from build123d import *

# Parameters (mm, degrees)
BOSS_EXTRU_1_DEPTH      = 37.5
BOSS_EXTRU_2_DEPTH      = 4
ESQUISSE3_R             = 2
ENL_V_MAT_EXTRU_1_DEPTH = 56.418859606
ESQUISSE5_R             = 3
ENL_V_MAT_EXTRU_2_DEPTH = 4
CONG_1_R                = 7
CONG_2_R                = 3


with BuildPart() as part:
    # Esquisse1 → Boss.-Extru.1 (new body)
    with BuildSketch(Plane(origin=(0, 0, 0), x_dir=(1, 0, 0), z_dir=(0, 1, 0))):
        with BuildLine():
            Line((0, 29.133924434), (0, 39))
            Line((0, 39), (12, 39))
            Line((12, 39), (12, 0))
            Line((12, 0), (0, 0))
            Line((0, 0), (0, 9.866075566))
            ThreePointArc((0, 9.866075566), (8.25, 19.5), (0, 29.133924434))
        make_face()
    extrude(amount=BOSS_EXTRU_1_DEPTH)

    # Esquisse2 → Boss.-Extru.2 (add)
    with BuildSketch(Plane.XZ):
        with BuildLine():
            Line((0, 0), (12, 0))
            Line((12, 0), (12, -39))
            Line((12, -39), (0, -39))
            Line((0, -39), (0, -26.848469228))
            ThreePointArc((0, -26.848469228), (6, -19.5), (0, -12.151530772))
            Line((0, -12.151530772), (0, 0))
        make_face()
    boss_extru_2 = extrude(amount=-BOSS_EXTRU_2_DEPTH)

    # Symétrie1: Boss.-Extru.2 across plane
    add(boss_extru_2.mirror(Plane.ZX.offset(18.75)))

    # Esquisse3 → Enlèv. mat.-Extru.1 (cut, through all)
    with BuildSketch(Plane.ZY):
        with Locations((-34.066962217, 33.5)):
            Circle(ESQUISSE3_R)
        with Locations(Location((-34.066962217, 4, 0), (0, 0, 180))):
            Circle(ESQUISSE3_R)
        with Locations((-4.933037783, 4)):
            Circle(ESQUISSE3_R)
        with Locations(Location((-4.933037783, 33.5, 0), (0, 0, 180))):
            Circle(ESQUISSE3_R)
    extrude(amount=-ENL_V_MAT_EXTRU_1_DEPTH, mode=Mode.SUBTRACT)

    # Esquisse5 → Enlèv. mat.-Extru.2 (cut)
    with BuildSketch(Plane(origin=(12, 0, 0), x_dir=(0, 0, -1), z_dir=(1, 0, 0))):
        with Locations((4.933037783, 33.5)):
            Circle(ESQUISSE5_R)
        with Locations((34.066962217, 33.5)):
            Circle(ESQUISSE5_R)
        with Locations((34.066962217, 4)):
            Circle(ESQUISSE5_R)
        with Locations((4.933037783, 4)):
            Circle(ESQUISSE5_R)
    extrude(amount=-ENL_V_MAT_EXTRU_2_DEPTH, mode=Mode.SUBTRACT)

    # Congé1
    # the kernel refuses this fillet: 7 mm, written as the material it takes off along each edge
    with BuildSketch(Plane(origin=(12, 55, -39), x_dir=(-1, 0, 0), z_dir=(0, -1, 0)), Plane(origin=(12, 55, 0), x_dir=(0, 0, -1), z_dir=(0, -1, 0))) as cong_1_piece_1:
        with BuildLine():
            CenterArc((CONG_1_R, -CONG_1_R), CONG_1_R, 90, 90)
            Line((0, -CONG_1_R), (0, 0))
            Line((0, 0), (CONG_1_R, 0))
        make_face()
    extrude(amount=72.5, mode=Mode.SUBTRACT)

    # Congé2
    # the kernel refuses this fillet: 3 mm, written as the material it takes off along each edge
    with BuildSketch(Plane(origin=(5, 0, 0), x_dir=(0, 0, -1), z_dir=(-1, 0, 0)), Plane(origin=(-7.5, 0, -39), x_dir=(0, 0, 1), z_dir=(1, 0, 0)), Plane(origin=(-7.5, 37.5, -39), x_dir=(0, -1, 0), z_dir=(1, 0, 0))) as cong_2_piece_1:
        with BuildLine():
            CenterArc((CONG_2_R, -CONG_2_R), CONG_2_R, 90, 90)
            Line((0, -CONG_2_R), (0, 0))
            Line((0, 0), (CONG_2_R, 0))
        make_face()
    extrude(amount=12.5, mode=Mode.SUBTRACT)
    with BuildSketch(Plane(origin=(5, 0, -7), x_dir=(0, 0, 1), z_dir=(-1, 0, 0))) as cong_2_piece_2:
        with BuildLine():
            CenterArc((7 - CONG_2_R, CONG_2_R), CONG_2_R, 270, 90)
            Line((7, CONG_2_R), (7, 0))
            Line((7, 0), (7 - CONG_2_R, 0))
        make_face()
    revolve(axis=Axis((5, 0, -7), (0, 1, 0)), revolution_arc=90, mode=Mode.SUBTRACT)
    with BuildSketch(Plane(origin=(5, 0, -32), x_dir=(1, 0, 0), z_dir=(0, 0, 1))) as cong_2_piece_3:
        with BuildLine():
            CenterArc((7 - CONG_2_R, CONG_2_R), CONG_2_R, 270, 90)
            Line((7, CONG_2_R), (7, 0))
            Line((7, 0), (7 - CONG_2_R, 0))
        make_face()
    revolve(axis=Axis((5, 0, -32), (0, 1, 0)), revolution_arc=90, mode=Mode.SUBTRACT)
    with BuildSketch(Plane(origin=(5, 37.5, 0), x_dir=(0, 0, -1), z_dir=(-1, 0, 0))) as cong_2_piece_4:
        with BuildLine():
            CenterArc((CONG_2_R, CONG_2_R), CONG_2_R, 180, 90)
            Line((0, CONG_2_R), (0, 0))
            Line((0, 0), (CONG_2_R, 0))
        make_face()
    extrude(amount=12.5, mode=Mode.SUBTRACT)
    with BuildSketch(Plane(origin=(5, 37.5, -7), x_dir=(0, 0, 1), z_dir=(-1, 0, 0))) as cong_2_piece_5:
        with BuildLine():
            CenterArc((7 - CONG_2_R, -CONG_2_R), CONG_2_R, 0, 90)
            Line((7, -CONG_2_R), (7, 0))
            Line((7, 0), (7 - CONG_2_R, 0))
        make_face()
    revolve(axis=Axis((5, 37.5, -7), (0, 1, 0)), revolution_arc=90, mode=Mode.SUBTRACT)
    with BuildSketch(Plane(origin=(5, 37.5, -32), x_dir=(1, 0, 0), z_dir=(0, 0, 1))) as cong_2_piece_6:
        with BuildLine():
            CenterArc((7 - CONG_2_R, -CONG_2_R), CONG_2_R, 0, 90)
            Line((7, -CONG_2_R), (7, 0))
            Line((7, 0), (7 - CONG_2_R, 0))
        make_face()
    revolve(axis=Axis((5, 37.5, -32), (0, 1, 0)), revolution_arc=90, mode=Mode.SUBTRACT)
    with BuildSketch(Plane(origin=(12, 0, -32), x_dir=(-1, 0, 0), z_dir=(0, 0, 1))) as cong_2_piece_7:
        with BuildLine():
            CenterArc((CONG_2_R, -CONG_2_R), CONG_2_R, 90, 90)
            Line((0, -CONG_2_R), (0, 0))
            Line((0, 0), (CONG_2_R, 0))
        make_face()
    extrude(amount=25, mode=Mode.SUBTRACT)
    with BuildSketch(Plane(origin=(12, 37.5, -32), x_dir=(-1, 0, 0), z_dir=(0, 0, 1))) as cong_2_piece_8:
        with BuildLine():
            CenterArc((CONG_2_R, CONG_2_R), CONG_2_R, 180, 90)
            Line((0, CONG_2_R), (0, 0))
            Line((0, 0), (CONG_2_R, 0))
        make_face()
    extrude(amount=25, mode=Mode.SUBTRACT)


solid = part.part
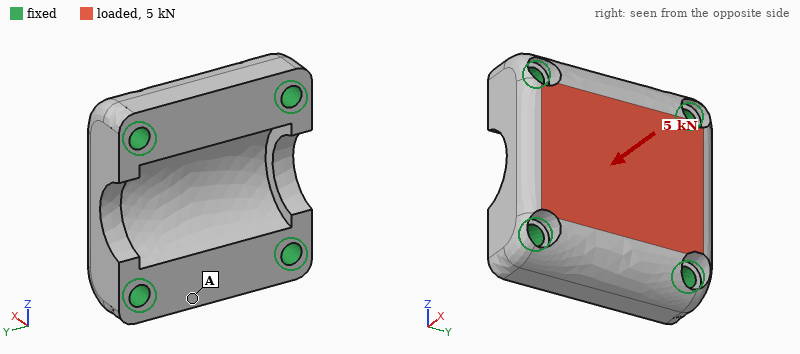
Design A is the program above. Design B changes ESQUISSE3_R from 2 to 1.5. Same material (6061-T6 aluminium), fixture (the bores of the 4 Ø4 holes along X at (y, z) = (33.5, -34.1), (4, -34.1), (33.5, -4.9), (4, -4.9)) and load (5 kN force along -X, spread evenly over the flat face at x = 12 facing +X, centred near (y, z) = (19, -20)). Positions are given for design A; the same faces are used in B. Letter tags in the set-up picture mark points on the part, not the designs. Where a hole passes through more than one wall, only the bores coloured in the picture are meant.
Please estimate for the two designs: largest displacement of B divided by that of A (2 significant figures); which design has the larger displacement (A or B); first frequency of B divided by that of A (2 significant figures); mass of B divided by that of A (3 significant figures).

1.1
B
0.93
1.02
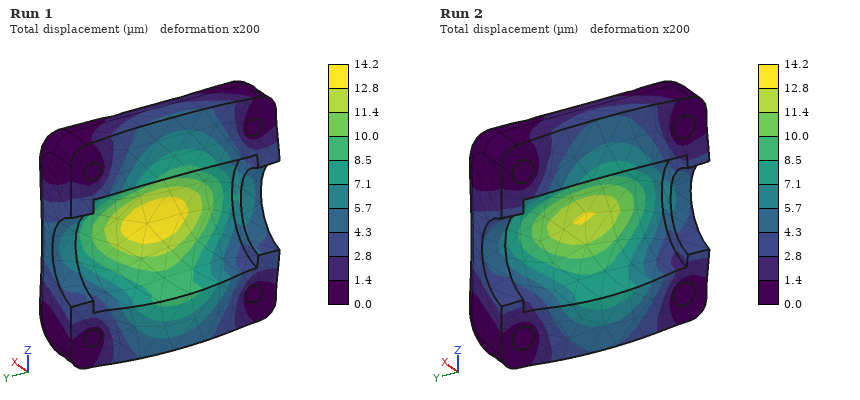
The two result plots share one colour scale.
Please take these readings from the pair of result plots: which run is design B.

Run 1
